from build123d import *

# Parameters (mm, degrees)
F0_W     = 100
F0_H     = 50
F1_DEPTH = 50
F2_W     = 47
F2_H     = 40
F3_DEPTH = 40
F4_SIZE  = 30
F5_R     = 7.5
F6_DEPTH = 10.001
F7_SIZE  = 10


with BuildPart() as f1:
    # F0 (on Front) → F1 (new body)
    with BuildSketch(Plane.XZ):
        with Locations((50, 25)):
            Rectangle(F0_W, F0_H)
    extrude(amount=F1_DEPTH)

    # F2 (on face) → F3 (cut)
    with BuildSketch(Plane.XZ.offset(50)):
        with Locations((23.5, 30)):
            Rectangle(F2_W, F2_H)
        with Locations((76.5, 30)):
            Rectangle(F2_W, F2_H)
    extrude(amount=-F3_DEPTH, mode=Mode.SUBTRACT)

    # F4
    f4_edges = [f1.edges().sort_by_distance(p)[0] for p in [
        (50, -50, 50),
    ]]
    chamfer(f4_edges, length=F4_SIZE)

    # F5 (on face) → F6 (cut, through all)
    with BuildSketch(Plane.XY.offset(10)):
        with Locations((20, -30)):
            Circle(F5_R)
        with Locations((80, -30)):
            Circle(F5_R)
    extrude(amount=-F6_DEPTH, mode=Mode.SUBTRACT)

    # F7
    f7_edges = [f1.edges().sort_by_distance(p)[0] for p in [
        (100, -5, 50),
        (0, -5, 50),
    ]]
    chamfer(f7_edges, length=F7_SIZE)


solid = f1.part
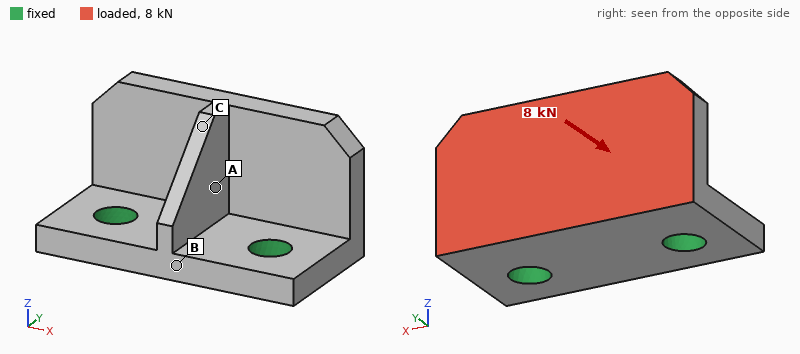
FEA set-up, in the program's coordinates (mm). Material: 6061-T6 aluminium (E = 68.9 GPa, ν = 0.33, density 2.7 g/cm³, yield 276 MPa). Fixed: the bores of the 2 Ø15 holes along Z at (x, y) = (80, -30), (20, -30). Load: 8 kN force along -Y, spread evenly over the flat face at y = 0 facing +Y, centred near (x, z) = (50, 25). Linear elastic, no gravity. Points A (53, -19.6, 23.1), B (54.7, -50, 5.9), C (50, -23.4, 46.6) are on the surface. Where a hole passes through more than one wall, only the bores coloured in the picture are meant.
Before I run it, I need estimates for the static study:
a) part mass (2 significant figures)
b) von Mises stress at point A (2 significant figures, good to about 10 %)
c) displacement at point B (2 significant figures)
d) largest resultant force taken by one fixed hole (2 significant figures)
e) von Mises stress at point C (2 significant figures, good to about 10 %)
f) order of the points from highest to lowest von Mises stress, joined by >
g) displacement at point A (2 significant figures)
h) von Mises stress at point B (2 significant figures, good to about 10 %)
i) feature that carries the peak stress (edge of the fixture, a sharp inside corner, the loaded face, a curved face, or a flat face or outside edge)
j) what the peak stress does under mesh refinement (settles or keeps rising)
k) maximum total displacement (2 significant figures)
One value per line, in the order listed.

250 g
24 MPa
0.044 mm
4.0 kN
11 MPa
B > A > C
0.052 mm
40 MPa
edge of the fixture
keeps rising
0.18 mm
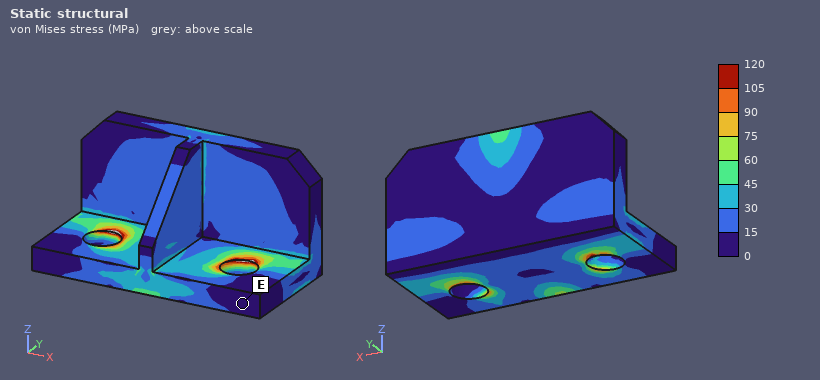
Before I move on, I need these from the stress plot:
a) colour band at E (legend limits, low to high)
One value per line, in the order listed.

0 to 15 MPa
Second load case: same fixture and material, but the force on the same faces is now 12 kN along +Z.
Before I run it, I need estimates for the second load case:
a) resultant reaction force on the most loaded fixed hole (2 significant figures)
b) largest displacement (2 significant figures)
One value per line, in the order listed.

6.0 kN
0.25 mm
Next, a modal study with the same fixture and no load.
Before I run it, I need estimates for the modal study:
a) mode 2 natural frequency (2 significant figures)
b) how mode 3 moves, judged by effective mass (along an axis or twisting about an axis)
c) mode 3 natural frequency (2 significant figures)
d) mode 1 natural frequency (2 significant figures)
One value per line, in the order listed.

4300 Hz
along X
6700 Hz
3200 Hz
